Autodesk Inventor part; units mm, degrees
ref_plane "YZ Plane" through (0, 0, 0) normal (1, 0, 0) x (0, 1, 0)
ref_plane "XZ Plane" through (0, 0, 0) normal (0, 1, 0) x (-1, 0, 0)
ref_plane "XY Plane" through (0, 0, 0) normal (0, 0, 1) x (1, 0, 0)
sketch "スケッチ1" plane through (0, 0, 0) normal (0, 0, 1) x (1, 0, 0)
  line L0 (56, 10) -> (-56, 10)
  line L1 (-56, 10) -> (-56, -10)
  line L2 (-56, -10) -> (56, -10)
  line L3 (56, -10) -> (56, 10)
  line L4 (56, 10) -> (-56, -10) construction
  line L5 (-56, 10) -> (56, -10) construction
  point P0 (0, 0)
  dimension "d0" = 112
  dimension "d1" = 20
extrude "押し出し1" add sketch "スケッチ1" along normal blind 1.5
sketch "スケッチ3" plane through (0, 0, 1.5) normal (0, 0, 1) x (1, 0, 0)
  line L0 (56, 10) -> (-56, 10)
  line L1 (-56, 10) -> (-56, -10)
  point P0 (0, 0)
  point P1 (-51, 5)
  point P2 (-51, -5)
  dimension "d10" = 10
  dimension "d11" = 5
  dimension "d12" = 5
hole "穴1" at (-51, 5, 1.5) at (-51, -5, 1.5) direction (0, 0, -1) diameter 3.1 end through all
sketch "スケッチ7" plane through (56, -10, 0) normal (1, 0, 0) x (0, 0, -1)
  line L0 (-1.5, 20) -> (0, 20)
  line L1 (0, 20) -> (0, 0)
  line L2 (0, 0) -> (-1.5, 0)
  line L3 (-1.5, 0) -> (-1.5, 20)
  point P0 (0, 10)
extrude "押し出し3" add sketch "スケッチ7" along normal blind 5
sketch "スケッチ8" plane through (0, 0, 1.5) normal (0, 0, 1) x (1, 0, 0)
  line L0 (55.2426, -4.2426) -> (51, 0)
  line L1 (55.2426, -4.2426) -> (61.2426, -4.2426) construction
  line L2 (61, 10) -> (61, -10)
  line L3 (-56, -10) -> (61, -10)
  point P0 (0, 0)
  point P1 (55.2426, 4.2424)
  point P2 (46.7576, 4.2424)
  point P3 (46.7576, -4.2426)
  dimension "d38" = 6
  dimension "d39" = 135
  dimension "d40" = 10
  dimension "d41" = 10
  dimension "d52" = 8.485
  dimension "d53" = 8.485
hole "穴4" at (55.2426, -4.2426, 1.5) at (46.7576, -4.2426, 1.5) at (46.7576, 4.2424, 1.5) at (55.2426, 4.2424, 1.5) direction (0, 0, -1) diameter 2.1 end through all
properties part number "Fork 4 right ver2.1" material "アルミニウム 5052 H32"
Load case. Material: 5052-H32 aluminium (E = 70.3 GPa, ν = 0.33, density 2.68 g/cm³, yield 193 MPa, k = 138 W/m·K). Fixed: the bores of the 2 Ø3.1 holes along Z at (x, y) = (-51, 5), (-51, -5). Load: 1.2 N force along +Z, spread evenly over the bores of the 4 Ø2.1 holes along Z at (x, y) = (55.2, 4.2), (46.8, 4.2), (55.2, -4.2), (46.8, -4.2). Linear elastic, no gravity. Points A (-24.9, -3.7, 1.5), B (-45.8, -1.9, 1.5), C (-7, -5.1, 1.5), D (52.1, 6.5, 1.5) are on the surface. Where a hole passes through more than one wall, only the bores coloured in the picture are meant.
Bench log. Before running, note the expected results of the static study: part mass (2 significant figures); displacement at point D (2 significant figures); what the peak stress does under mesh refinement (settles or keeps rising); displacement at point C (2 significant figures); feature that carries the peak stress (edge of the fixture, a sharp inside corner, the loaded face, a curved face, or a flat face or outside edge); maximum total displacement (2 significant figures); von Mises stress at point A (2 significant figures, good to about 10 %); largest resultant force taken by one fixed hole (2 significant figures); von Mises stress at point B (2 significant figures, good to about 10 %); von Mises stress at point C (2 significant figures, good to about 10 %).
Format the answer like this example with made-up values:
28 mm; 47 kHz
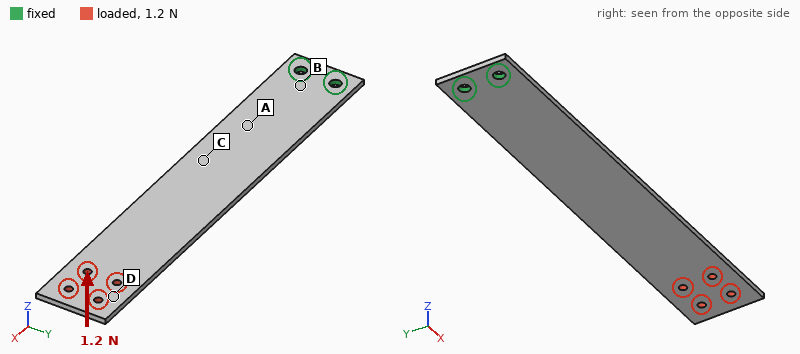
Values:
9.3 g; 1.0 mm; keeps rising; 0.24 mm; edge of the fixture; 1.2 mm; 12 MPa; 0.61 N; 14 MPa; 9.3 MPa
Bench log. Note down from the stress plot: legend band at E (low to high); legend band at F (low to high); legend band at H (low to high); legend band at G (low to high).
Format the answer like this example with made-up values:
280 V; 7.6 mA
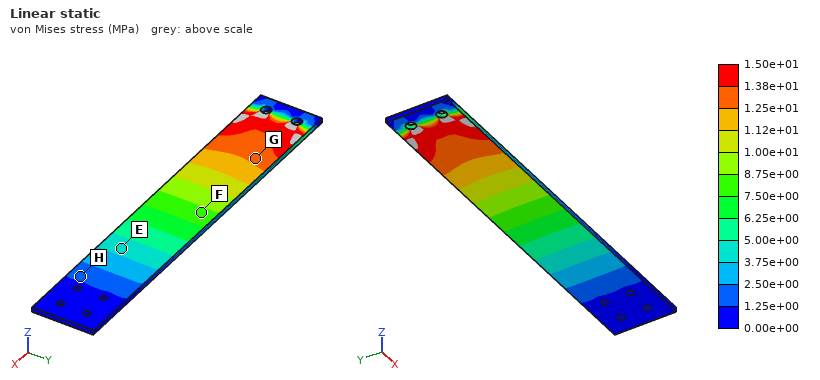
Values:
3.75e+00 to 5.00e+00 MPa; 7.50e+00 to 8.75e+00 MPa; 1.25e+00 to 2.50e+00 MPa; 1.25e+01 to 1.38e+01 MPa
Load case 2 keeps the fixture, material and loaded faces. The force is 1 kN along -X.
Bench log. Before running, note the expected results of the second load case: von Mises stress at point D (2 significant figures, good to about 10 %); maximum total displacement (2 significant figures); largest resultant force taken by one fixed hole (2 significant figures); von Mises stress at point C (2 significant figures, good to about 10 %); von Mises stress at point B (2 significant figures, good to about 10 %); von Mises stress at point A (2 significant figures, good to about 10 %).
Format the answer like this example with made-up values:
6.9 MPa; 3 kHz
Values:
20 MPa; 50 µm; 500 N; 33 MPa; 32 MPa; 33 MPa
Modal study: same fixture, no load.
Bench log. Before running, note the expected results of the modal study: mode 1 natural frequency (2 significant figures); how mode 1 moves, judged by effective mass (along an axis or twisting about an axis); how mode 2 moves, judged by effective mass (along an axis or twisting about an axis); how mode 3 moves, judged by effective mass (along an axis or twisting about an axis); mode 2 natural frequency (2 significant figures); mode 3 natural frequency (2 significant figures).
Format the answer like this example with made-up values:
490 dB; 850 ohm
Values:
100 Hz; along Z; along Z; twisting about X; 640 Hz; 1100 Hz
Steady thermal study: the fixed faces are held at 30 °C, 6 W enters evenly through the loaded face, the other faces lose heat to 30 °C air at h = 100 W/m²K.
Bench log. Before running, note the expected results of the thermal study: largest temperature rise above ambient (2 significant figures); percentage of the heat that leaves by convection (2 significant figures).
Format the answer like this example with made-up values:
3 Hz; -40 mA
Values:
35 K; 94 %
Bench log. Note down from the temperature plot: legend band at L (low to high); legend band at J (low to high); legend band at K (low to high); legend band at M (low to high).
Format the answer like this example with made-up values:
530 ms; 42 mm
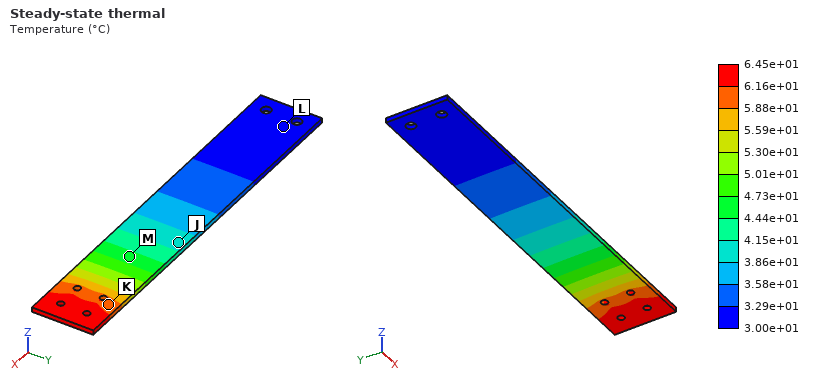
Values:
3.00e+01 to 3.29e+01 °C; 3.86e+01 to 4.15e+01 °C; 5.88e+01 to 6.16e+01 °C; 4.44e+01 to 4.73e+01 °C
